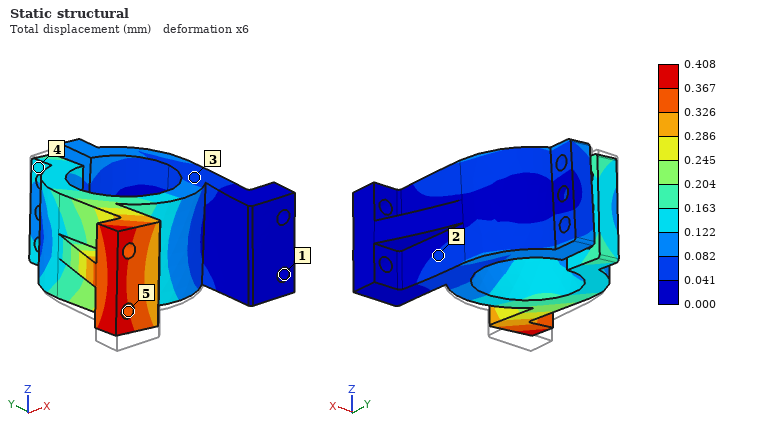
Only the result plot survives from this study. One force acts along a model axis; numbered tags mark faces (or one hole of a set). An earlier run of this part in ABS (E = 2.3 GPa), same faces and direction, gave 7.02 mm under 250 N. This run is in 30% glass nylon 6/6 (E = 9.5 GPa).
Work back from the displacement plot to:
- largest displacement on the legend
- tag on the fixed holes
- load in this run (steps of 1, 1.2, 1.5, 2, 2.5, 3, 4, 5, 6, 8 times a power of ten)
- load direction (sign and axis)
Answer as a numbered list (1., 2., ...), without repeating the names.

1. 0.408 mm
2. 1
3. 60 N
4. +Z
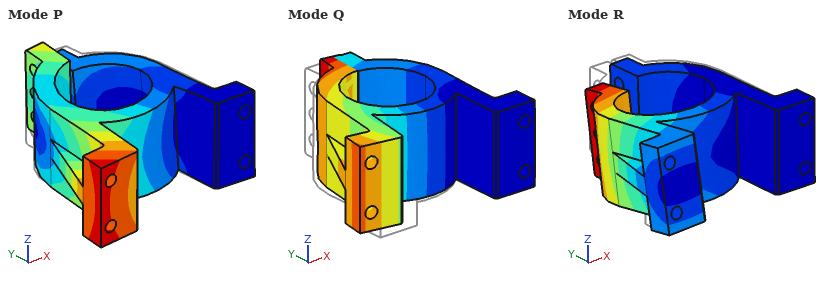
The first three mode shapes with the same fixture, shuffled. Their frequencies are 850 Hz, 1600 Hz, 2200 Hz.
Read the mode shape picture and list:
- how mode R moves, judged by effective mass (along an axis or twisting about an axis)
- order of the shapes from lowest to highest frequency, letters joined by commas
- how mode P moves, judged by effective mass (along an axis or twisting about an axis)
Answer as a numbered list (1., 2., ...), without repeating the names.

1. along Z
2. Q, R, P
3. along Z
